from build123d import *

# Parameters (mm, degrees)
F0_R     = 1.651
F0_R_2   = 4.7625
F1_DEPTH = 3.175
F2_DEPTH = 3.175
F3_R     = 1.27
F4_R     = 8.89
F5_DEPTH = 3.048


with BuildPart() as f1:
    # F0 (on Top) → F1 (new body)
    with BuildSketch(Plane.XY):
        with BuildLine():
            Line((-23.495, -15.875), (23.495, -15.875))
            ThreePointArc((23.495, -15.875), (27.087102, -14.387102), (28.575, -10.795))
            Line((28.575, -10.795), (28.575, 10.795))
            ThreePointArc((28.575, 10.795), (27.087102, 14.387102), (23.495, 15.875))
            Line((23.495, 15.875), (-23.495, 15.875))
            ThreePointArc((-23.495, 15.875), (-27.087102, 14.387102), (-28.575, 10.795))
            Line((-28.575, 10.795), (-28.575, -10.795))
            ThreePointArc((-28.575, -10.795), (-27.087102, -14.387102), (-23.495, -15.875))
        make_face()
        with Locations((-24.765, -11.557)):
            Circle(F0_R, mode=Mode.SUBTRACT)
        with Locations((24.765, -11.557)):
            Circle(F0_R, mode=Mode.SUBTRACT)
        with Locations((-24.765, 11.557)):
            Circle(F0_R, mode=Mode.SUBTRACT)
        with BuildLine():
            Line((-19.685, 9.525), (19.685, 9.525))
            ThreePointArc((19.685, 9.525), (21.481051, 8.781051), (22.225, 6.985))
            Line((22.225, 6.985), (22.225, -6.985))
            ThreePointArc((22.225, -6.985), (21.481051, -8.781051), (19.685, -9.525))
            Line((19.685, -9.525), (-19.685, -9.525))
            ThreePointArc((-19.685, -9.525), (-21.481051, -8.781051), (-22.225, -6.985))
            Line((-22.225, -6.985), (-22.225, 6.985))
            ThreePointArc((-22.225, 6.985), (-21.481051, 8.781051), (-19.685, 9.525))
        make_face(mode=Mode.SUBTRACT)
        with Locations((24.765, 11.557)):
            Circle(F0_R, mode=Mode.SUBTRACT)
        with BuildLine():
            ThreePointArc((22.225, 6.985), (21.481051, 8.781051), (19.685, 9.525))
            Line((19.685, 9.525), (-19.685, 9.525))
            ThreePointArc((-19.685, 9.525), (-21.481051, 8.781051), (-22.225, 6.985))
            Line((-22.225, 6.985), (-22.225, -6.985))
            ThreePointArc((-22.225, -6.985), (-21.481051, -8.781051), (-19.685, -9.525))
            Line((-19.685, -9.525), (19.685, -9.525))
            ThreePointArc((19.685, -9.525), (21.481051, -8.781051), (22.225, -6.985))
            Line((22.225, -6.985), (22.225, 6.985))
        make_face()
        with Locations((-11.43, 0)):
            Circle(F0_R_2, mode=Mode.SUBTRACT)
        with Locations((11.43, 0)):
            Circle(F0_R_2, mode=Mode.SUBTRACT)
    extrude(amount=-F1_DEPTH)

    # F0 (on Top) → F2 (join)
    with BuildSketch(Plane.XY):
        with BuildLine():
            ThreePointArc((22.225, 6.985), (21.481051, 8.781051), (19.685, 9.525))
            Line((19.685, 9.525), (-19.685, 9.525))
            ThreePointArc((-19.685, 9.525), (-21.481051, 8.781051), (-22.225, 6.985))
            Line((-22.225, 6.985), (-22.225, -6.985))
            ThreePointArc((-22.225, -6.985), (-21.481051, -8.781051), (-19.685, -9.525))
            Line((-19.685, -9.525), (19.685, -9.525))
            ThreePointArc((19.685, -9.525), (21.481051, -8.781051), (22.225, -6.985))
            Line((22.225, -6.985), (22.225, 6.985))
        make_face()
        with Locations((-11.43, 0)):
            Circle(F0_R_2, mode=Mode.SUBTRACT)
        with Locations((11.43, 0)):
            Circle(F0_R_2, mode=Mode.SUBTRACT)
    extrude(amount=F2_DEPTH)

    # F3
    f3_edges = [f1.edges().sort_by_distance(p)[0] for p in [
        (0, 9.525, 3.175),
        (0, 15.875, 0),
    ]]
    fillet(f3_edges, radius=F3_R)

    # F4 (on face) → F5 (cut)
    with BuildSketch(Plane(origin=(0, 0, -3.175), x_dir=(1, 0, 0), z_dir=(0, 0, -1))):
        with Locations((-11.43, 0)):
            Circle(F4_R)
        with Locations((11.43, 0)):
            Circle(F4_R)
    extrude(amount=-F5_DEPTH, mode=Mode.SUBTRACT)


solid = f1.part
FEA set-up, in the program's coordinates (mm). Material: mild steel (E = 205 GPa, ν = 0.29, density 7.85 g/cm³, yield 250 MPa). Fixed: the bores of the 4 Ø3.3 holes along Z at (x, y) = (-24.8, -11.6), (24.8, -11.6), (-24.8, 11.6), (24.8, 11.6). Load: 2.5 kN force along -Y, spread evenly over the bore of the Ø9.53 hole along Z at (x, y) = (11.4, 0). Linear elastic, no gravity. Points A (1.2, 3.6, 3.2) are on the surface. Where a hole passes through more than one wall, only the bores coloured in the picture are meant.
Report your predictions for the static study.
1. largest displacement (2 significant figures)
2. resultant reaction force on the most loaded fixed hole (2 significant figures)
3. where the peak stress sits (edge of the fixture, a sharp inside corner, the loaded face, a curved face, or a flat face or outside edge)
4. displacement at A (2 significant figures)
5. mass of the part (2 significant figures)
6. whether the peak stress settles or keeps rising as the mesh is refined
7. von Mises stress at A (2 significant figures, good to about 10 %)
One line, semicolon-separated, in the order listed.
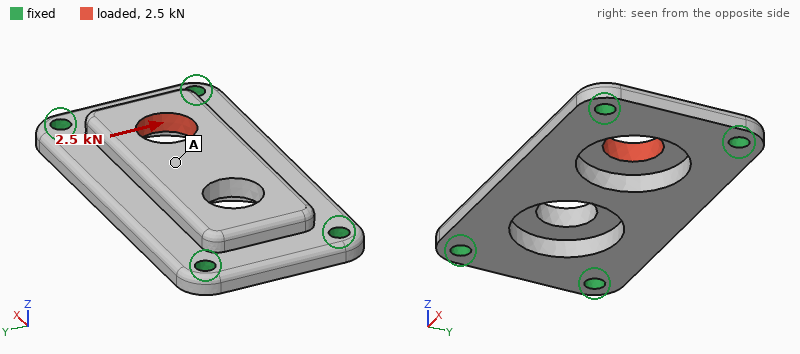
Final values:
6.6 µm; 1.1 kN; edge of the fixture; 5.1 µm; 48 g; keeps rising; 15 MPa
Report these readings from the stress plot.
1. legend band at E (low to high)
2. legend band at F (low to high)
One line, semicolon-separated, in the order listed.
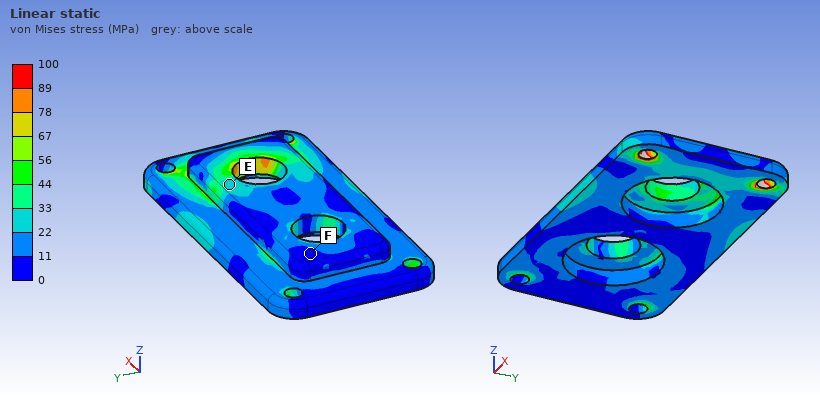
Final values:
22 to 33 MPa; 0 to 11 MPa
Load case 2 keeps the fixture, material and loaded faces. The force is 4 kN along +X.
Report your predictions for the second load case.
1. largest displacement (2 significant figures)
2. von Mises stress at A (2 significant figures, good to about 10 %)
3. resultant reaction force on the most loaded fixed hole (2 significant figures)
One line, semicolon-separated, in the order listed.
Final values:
8.5 µm; 38 MPa; 1.2 kN
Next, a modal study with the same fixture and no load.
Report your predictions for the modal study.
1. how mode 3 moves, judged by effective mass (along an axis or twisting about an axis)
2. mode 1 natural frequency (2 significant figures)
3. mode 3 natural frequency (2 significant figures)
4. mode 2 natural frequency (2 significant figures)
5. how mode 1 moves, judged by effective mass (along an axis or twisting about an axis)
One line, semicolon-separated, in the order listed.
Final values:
along Y; 8100 Hz; 20 kHz; 11 kHz; along Z
